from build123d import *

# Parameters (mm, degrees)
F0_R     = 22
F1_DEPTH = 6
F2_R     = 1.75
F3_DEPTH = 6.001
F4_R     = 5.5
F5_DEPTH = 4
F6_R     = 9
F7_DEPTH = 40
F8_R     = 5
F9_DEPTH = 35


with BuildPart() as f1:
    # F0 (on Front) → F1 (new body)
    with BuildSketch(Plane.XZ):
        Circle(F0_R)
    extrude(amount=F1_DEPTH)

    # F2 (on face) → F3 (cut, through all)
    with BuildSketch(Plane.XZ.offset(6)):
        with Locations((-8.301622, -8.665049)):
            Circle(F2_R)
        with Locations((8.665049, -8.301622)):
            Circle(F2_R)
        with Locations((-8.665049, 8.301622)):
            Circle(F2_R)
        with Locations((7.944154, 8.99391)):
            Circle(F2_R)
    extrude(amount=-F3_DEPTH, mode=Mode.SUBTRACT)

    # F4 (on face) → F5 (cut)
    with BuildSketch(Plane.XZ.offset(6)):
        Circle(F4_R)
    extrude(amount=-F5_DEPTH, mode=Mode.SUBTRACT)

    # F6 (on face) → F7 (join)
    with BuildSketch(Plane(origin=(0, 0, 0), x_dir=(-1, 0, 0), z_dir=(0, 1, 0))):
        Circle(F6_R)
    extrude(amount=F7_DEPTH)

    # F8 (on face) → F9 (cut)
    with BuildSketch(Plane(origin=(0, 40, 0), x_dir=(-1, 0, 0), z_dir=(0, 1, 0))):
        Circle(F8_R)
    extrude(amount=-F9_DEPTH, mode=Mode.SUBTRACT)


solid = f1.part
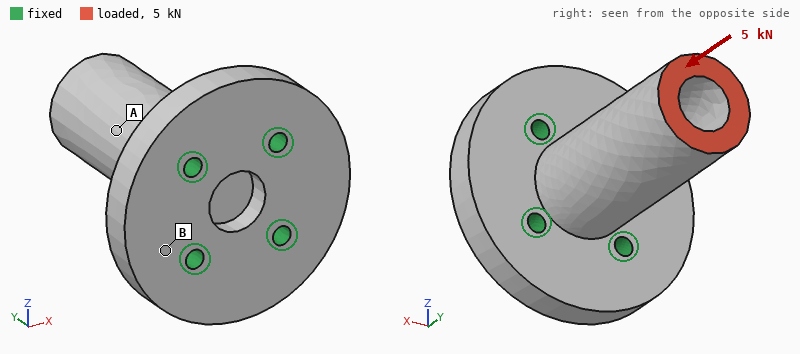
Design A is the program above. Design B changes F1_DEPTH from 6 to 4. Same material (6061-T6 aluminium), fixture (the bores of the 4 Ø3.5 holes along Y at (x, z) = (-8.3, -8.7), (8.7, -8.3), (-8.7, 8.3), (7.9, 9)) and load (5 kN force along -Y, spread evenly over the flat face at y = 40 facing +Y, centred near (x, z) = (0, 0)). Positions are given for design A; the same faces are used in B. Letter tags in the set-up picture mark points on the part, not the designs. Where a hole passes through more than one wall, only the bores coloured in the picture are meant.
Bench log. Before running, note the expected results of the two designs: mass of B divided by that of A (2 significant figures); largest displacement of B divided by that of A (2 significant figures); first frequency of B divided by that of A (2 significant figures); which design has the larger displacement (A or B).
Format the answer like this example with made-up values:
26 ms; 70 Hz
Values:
0.83; 1.1; 0.92; B
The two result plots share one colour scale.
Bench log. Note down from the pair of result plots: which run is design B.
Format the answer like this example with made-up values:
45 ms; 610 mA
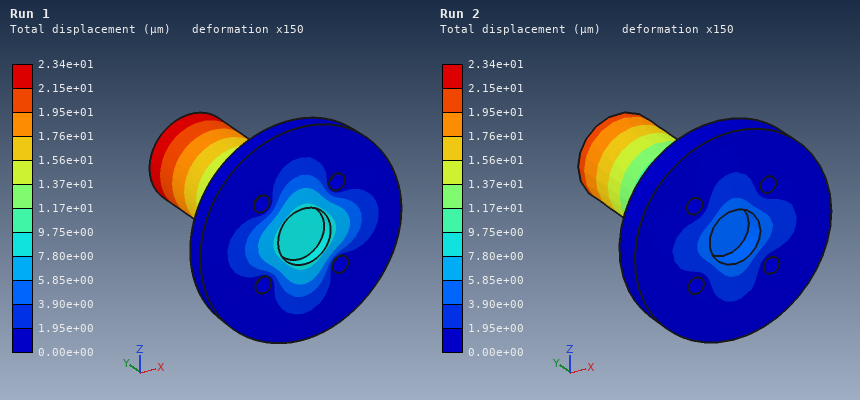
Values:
Run 1
